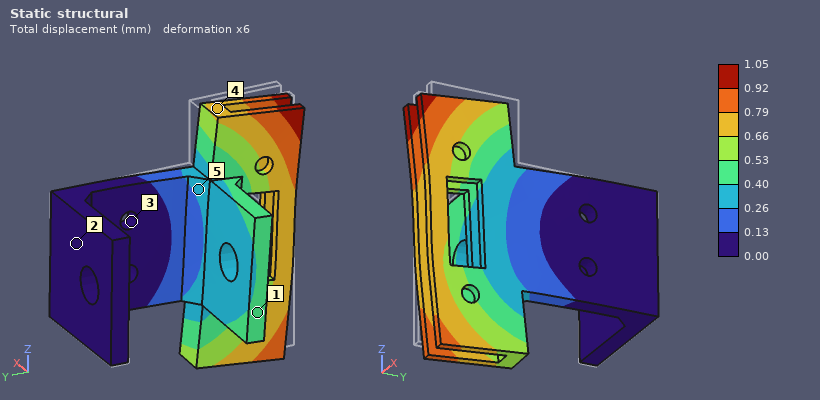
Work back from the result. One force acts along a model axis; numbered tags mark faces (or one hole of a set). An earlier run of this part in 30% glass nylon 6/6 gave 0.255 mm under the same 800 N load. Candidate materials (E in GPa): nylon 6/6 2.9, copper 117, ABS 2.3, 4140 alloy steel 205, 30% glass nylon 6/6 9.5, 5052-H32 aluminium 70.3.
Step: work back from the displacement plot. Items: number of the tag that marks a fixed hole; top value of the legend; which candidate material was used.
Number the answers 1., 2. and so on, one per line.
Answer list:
1. 3
2. 1.05 mm
3. ABS
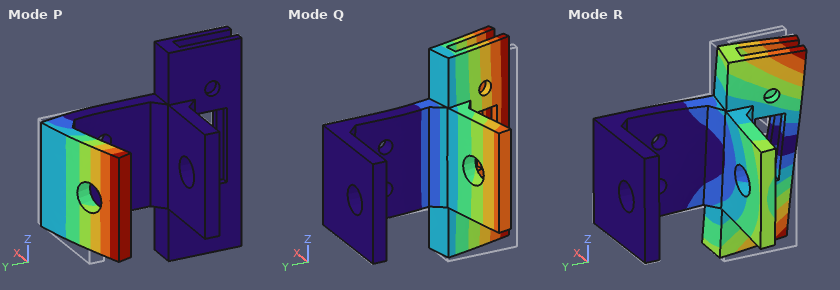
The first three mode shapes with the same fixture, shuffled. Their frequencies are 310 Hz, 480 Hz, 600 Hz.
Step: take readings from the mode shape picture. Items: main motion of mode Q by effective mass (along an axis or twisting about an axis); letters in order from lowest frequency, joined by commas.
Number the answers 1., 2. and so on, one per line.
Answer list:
1. along X
2. Q, R, P
